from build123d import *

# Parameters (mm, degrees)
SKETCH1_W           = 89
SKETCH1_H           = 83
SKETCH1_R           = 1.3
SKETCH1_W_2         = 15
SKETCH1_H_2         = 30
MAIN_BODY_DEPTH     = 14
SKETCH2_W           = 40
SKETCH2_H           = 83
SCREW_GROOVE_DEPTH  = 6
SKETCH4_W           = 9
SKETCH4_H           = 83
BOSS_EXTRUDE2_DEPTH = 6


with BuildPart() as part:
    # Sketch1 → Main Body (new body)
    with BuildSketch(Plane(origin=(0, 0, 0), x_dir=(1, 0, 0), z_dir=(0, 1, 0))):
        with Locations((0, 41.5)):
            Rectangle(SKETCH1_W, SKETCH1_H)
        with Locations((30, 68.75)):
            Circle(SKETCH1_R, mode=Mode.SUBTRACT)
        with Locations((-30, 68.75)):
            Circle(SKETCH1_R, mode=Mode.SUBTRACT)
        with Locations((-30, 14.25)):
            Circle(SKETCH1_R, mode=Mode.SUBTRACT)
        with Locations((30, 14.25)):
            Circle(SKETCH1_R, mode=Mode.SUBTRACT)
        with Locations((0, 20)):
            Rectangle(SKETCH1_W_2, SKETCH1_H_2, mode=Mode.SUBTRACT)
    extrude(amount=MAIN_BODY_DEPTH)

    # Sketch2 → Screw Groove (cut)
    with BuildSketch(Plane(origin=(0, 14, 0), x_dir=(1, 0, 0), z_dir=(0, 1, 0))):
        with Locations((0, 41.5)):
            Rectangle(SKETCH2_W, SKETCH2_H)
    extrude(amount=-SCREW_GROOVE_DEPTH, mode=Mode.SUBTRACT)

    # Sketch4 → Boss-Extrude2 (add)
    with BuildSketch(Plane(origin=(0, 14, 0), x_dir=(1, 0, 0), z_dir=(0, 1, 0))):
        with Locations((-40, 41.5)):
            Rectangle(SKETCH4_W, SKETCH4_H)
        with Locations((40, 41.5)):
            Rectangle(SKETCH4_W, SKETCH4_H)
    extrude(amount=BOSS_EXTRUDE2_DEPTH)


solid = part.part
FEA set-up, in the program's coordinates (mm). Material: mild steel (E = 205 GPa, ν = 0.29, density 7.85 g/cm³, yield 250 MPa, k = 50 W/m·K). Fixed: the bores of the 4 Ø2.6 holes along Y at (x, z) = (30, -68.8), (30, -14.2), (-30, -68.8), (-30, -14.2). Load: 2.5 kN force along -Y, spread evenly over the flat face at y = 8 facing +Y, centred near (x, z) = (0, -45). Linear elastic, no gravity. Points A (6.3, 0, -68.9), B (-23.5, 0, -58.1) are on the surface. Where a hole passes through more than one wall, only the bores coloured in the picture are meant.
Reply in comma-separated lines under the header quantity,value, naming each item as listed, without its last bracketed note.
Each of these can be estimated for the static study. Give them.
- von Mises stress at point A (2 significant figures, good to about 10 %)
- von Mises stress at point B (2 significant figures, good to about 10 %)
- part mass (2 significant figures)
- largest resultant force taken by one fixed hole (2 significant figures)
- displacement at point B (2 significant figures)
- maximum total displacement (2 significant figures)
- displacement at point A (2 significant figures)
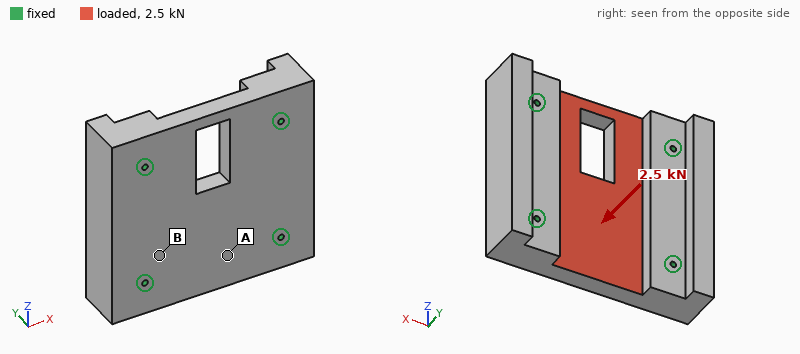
quantity,value
von Mises stress at point A,9.1 MPa
von Mises stress at point B,3.1 MPa
part mass,700 g
largest resultant force taken by one fixed hole,810 N
displacement at point B,1.1 µm
maximum total displacement,3.8 µm
displacement at point A,2.8 µm
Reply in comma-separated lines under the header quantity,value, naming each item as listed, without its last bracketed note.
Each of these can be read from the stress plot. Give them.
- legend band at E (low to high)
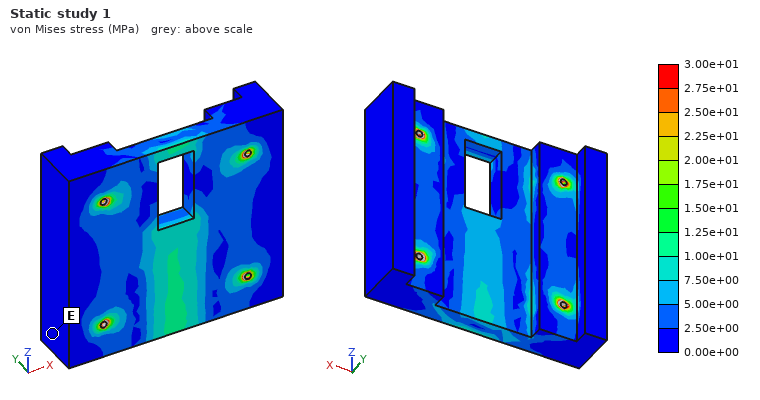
quantity,value
legend band at E,0.00e+00 to 2.50e+00 MPa
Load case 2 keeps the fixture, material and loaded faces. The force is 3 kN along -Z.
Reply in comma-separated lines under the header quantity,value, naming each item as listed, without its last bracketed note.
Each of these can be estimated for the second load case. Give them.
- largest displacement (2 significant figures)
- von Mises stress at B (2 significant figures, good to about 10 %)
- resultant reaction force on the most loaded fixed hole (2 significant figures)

quantity,value
largest displacement,1.5 µm
von Mises stress at B,3.0 MPa
resultant reaction force on the most loaded fixed hole,800 N
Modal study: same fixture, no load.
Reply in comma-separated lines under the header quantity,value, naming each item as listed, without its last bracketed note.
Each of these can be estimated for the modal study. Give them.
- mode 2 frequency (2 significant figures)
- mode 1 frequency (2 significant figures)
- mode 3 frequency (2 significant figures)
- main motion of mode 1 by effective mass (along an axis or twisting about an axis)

quantity,value
mode 2 frequency,13 kHz
mode 1 frequency,10 kHz
mode 3 frequency,13 kHz
main motion of mode 1 by effective mass,along Y
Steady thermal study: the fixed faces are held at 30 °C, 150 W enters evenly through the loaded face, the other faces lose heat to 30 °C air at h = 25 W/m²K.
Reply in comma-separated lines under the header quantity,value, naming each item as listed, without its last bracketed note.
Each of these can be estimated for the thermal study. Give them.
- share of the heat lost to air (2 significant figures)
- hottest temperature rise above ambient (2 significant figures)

quantity,value
share of the heat lost to air,7.0 %
hottest temperature rise above ambient,59 K
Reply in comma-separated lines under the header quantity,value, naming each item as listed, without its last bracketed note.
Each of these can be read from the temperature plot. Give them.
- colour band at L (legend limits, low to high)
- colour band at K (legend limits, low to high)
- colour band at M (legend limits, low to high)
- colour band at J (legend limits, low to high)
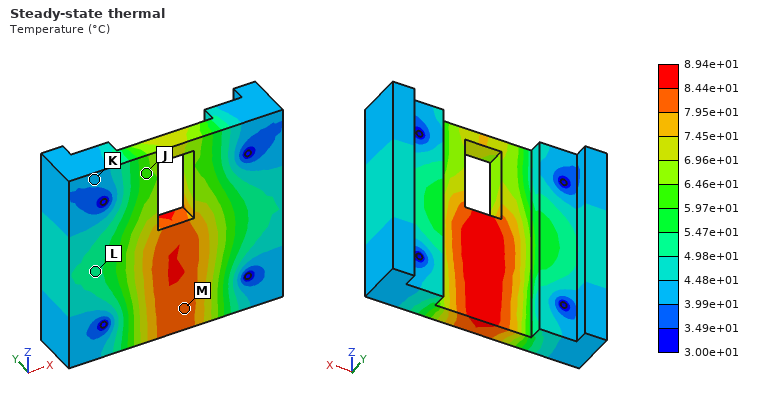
quantity,value
colour band at L,4.98e+01 to 5.47e+01 °C
colour band at K,3.99e+01 to 4.48e+01 °C
colour band at M,7.95e+01 to 8.44e+01 °C
colour band at J,5.97e+01 to 6.46e+01 °C
